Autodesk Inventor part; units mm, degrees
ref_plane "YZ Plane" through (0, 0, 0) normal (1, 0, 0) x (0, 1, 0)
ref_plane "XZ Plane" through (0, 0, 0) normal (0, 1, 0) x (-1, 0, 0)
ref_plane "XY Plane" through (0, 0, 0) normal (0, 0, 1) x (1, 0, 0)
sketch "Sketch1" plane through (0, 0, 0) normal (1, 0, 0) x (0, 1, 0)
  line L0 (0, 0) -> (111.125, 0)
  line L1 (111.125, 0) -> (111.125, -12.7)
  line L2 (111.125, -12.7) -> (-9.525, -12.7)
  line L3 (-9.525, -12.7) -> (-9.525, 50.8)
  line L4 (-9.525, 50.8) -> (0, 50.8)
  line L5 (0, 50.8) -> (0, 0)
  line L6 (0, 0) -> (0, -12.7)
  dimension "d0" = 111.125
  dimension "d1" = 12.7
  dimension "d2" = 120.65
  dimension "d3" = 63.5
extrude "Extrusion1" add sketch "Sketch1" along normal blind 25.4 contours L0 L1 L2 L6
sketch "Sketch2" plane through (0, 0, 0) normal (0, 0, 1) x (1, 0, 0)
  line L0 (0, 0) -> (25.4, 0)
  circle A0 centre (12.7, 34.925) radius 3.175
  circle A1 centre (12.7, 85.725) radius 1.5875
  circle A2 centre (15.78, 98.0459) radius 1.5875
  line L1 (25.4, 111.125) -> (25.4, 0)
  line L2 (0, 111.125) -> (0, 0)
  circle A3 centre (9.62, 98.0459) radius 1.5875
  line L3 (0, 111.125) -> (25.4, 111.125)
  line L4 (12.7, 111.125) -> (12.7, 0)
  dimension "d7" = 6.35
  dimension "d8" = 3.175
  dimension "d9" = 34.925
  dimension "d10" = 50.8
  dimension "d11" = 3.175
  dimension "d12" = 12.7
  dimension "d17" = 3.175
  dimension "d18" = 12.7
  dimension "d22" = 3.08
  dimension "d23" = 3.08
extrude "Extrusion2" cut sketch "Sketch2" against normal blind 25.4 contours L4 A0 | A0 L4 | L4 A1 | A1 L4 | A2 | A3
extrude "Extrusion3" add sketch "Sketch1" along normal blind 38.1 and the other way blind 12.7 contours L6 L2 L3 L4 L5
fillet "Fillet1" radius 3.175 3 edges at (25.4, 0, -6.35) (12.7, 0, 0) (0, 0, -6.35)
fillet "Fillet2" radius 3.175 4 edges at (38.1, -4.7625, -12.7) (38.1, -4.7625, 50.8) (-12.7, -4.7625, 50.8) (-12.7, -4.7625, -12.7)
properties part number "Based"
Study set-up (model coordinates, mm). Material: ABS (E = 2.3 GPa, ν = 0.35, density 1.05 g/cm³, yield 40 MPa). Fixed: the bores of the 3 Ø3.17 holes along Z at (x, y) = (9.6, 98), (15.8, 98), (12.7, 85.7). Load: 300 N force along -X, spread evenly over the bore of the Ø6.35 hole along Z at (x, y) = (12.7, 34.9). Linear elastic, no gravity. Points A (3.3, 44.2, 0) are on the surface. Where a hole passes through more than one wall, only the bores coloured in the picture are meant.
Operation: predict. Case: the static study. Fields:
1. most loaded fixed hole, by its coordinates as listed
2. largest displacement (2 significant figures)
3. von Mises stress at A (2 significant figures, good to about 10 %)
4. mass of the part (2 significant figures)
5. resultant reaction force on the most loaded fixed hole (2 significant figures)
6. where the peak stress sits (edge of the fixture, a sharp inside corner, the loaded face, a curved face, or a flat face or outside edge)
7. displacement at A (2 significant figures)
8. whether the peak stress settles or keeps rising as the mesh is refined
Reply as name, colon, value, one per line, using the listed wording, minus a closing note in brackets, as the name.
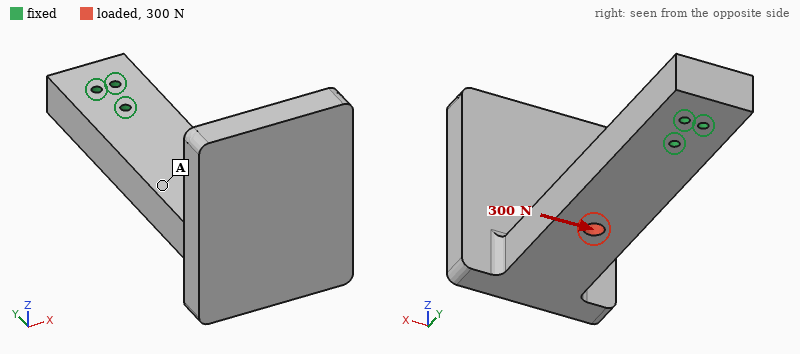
most loaded fixed hole, by its coordinates as listed: (12.7, 85.7)
largest displacement: 1.4 mm
von Mises stress at A: 1.9 MPa
mass of the part: 69 g
resultant reaction force on the most loaded fixed hole: 1.0 kN
where the peak stress sits: edge of the fixture
displacement at A: 0.53 mm
whether the peak stress settles or keeps rising as the mesh is refined: keeps rising
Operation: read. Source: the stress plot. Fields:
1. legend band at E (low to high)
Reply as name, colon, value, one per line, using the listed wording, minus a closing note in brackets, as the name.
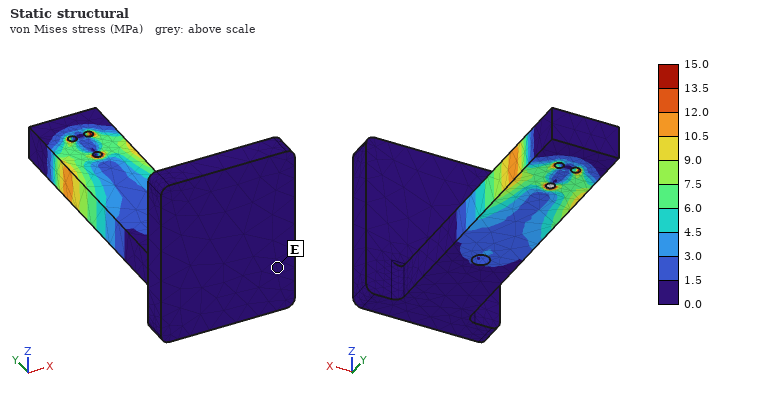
legend band at E: 0.0 to 1.5 MPa
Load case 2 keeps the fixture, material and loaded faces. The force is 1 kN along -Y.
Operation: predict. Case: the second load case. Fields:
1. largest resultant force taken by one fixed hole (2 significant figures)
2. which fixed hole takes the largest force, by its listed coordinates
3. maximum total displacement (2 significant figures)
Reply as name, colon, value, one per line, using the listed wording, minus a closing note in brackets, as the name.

largest resultant force taken by one fixed hole: 640 N
which fixed hole takes the largest force, by its listed coordinates: (12.7, 85.7)
maximum total displacement: 91 µm
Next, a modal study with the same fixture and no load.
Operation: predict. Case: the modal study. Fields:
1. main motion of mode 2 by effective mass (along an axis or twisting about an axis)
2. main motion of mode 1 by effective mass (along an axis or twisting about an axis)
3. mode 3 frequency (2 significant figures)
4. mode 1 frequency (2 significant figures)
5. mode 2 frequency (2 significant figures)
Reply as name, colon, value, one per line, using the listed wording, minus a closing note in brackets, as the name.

main motion of mode 2 by effective mass: along X
main motion of mode 1 by effective mass: along Z
mode 3 frequency: 440 Hz
mode 1 frequency: 140 Hz
mode 2 frequency: 200 Hz
